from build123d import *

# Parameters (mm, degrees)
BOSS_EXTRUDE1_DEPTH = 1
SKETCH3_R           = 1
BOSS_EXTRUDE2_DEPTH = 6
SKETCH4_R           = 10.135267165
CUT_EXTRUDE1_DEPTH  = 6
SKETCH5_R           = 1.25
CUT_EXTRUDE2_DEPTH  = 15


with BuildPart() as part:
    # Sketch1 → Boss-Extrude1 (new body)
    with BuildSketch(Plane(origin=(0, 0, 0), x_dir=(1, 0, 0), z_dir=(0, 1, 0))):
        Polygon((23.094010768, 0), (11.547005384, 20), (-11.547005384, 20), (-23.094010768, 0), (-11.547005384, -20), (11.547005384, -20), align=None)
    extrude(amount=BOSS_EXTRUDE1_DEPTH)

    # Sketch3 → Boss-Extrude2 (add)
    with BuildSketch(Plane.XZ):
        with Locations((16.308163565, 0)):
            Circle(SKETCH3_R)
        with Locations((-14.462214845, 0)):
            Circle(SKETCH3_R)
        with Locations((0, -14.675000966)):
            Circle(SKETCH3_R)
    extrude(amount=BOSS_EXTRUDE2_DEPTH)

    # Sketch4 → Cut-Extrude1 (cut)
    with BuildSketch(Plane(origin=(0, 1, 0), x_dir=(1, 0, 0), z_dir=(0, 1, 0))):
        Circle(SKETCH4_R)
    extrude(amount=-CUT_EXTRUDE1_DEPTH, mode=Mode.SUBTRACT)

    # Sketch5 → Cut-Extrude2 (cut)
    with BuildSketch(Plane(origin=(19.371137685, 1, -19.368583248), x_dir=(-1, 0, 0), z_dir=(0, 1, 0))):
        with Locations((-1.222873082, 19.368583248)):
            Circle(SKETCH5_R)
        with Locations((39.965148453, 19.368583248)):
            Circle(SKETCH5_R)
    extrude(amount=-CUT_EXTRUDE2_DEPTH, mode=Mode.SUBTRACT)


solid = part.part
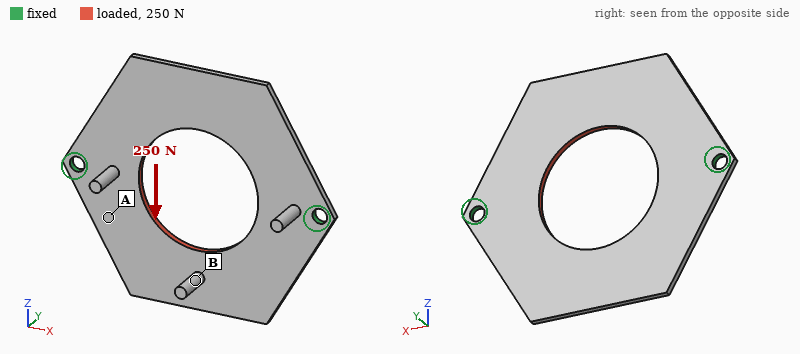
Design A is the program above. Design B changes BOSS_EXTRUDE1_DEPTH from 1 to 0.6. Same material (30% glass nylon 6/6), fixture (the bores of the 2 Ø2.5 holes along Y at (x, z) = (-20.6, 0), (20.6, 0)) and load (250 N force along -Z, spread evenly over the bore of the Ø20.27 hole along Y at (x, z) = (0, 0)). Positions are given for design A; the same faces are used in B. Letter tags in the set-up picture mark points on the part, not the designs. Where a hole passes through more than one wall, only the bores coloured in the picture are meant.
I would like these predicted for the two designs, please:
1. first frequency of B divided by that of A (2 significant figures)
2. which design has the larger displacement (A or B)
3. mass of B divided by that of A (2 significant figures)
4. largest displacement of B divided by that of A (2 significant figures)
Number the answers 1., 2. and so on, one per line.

1. 0.61
2. B
3. 0.62
4. 1.7
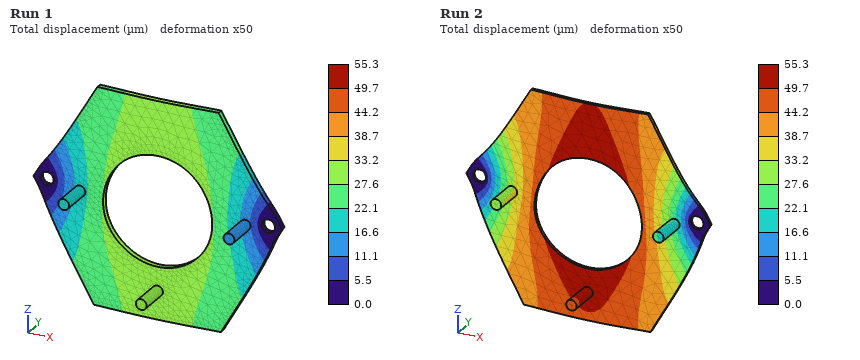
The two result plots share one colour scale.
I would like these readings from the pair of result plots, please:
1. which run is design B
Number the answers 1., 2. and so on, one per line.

1. Run 2
